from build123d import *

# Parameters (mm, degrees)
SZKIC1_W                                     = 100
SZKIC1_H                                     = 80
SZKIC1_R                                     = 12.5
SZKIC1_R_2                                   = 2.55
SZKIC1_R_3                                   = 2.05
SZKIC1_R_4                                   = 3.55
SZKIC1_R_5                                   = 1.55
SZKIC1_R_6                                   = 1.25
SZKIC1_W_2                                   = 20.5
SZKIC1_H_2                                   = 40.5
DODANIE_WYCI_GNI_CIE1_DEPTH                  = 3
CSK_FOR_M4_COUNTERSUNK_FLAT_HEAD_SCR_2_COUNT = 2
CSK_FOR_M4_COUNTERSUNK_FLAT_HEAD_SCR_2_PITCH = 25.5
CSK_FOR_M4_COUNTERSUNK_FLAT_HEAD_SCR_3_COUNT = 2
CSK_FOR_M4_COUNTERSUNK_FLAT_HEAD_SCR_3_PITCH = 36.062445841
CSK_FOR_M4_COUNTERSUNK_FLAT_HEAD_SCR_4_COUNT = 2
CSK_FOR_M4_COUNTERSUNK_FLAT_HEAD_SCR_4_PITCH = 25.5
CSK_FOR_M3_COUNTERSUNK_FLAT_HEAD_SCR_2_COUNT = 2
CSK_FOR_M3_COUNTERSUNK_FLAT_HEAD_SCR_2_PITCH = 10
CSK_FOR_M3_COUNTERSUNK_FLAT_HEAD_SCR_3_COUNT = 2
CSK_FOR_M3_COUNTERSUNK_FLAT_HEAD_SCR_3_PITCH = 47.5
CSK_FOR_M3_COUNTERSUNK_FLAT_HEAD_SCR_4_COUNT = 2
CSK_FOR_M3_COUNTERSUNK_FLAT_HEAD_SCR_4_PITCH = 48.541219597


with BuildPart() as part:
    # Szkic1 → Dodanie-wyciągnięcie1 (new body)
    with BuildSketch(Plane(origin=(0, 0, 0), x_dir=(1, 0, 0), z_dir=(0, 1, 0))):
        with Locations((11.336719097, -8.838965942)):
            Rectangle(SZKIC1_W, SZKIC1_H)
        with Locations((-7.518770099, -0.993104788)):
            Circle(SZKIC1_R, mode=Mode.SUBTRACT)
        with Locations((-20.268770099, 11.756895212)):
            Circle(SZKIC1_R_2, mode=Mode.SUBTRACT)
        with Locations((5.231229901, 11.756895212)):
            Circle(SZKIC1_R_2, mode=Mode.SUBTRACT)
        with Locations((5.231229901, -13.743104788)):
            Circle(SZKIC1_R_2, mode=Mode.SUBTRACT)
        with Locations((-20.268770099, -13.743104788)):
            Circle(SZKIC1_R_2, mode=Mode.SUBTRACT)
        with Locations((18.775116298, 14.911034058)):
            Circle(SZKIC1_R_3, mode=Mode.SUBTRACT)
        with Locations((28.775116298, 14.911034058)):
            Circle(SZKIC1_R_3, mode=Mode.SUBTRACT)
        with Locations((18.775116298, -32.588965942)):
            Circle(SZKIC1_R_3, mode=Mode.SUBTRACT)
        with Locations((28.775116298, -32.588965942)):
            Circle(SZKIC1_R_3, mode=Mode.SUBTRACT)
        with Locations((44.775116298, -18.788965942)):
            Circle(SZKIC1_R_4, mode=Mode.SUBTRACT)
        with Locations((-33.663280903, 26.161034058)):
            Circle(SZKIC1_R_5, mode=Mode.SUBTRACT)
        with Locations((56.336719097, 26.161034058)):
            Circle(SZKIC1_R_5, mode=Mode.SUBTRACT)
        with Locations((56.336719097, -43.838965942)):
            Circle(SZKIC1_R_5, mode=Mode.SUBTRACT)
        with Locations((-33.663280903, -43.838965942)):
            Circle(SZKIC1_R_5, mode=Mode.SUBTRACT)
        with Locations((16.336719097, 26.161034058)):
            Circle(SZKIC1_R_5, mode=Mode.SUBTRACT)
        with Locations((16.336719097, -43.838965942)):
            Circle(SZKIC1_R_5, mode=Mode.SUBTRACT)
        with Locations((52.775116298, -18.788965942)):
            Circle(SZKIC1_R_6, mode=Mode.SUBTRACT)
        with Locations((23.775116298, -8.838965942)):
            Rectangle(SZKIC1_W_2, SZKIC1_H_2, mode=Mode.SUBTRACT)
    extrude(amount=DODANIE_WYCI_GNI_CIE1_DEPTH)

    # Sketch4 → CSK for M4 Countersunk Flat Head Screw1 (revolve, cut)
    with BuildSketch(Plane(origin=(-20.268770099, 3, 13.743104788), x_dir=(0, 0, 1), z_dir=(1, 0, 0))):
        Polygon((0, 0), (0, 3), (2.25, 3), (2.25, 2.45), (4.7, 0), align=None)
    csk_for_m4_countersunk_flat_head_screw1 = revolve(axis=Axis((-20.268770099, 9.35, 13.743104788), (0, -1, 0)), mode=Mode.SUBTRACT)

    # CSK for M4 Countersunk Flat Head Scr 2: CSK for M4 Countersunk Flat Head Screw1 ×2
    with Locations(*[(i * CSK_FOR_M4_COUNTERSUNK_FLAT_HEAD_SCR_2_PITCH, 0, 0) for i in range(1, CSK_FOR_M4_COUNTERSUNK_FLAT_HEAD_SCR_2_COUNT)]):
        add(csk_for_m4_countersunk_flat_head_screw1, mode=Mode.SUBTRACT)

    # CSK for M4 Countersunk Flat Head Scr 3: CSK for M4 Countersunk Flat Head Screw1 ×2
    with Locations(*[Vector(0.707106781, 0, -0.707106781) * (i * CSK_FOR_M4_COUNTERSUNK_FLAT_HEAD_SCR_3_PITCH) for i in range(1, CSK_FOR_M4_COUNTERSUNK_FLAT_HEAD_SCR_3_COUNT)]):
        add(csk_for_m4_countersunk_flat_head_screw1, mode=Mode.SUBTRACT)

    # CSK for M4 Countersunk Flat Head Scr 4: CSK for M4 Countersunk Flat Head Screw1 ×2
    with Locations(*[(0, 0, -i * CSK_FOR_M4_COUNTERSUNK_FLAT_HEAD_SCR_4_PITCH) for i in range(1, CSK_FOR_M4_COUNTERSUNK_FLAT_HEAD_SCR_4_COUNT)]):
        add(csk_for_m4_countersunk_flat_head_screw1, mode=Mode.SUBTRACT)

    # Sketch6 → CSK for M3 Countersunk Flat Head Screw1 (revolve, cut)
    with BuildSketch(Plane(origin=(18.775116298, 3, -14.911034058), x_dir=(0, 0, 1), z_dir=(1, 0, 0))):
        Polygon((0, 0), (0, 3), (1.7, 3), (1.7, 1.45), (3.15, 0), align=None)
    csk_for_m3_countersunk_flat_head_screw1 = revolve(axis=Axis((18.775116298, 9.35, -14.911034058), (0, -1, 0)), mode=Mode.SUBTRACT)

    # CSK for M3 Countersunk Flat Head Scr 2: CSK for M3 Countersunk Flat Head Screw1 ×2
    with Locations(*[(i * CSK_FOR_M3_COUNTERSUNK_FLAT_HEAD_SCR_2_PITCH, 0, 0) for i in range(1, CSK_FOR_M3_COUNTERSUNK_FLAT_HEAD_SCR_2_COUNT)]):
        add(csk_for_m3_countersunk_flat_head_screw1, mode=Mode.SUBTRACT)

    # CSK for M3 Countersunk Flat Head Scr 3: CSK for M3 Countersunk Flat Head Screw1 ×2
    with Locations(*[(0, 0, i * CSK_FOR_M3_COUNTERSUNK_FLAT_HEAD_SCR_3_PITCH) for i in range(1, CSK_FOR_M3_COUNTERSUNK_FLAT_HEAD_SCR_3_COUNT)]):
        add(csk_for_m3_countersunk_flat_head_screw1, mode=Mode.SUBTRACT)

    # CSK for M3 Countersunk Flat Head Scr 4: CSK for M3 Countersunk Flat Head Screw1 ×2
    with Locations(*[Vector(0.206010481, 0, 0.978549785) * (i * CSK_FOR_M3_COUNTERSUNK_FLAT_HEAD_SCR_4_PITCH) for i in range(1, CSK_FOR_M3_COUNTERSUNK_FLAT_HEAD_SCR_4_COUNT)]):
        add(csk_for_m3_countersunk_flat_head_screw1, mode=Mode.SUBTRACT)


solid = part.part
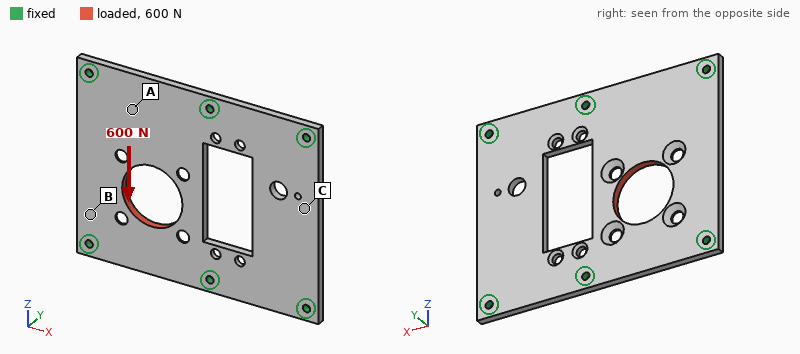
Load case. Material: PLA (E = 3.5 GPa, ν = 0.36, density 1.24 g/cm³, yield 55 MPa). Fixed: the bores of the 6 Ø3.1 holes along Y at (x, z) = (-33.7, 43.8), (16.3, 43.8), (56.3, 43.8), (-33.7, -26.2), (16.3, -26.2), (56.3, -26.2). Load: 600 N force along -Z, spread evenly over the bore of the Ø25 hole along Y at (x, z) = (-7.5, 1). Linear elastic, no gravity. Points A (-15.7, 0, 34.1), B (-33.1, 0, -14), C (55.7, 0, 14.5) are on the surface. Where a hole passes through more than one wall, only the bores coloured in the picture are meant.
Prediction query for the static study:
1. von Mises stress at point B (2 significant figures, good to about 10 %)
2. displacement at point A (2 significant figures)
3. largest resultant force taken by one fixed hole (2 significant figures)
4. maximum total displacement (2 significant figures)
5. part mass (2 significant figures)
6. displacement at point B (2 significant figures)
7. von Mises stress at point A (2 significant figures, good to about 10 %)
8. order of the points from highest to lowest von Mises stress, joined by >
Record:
3.1 MPa
24 µm
190 N
60 µm
24 g
15 µm
1.7 MPa
B > A > C
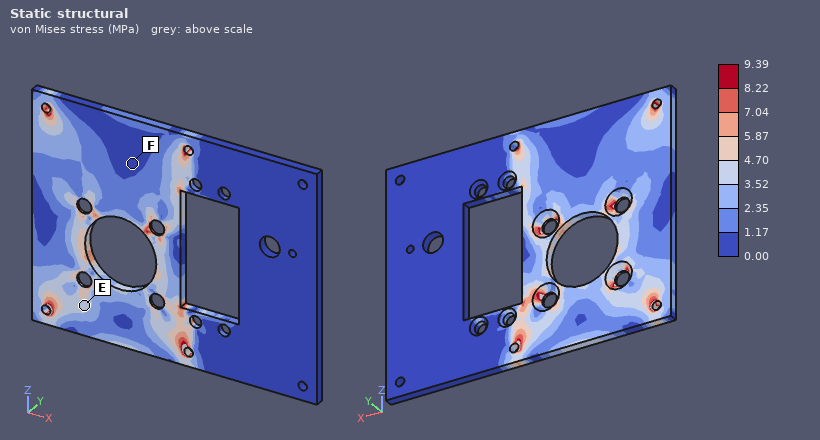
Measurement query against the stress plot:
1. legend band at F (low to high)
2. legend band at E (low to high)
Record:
0.00 to 1.17 MPa
3.52 to 4.70 MPa
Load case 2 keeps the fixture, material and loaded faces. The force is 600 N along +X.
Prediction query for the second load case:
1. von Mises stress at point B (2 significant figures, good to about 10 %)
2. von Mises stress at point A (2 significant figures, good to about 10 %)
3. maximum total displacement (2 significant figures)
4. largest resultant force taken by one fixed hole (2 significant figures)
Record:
2.5 MPa
2.7 MPa
98 µm
170 N
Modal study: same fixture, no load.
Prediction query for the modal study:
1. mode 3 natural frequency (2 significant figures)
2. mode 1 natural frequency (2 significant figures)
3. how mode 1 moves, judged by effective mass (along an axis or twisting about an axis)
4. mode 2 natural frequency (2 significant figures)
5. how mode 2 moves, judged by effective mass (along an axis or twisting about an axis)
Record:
1400 Hz
890 Hz
along Y
980 Hz
along Y
